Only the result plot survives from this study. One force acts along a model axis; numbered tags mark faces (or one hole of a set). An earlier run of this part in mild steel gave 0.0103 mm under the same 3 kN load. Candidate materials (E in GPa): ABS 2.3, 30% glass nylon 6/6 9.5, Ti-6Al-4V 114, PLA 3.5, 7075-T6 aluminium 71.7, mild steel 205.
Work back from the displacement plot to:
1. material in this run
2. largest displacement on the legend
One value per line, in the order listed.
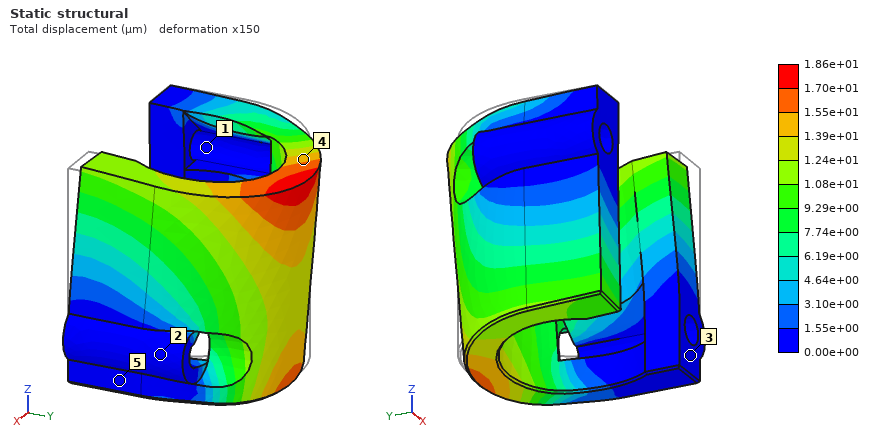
Ti-6Al-4V
1.86e+01 µm
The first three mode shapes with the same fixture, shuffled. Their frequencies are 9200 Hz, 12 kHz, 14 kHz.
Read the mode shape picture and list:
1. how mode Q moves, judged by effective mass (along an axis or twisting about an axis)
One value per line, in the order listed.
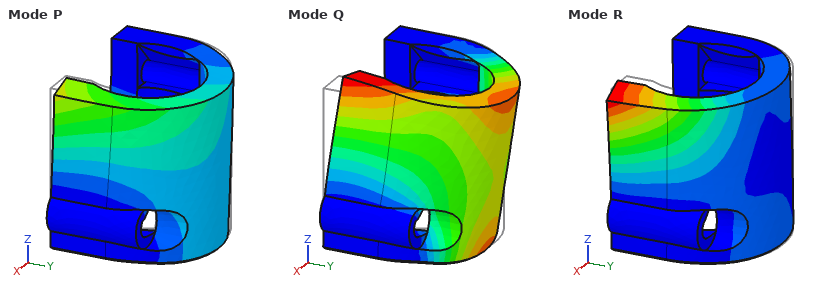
along X
